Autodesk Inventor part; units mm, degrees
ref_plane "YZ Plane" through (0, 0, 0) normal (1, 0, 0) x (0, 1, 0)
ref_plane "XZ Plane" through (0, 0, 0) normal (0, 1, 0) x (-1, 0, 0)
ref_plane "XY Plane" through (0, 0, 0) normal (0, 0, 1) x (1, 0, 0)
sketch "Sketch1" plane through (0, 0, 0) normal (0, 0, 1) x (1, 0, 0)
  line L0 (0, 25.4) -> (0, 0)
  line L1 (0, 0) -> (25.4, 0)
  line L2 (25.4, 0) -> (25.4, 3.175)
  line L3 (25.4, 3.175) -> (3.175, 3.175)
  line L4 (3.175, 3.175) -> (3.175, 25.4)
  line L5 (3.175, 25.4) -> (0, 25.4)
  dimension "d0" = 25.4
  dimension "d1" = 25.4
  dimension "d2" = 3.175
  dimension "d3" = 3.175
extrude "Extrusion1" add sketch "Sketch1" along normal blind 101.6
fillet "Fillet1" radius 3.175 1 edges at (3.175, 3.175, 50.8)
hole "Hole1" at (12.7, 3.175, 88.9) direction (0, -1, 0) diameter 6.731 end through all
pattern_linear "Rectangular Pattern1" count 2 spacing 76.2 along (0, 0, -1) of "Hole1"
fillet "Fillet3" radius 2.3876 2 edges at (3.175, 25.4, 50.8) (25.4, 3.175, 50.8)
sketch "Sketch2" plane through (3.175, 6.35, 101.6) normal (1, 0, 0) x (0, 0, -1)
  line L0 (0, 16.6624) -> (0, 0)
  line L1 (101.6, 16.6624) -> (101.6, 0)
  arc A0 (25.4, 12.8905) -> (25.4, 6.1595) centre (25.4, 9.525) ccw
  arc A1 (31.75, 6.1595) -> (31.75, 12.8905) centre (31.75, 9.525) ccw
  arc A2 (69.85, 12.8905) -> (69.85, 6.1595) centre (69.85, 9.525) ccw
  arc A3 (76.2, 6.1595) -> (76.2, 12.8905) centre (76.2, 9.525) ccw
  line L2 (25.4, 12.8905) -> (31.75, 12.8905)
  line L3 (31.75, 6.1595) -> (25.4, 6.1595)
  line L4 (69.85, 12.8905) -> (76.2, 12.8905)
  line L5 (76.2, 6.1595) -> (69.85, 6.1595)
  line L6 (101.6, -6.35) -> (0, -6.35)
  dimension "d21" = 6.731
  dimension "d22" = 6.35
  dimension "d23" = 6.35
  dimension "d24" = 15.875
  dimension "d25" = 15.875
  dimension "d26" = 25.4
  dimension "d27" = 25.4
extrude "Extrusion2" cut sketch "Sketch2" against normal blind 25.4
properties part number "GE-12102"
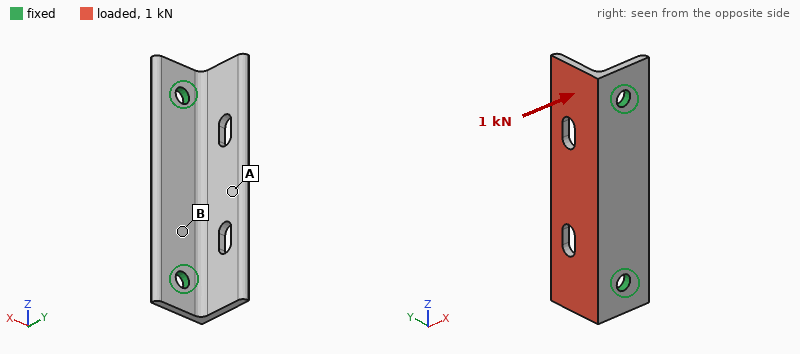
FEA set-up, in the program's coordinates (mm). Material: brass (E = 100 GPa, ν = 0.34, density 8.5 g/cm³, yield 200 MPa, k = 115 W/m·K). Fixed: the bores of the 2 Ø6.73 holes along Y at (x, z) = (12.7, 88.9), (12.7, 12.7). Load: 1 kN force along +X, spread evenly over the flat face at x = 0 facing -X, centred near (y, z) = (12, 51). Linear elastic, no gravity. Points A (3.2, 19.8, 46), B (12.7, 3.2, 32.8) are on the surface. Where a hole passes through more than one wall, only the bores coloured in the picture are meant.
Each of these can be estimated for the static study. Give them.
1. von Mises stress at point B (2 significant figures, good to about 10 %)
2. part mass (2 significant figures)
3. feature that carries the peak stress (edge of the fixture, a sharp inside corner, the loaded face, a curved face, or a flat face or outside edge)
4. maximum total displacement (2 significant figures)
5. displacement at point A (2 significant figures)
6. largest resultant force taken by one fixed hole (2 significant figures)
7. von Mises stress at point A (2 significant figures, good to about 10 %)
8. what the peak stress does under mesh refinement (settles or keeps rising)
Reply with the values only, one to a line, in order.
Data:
37 MPa
120 g
edge of the fixture
0.18 mm
0.13 mm
500 N
13 MPa
keeps rising
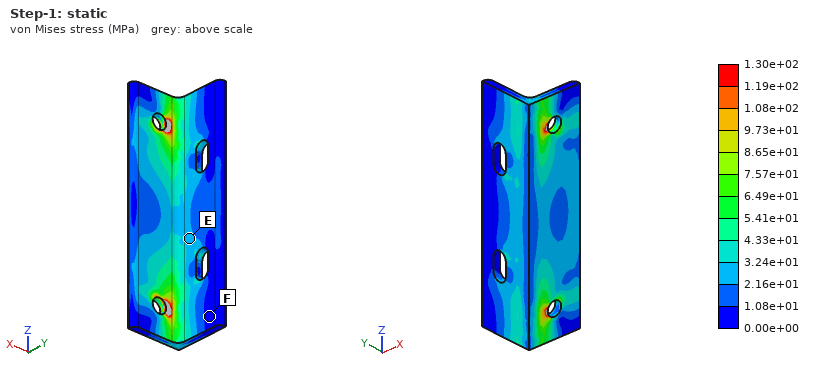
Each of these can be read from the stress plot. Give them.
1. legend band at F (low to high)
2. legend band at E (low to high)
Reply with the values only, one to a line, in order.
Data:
0.00e+00 to 1.08e+01 MPa
2.16e+01 to 3.24e+01 MPa
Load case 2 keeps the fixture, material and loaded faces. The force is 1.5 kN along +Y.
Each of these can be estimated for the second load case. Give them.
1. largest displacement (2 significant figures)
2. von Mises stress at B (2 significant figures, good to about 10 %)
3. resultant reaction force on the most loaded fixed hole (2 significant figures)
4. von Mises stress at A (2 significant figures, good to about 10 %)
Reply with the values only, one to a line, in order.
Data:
0.14 mm
26 MPa
790 N
14 MPa
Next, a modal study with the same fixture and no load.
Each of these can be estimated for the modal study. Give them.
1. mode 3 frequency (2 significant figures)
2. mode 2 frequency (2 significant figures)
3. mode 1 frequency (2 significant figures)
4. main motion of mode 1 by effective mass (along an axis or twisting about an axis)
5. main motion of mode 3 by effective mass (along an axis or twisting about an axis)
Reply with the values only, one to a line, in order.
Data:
3200 Hz
2600 Hz
1800 Hz
along X
along Y
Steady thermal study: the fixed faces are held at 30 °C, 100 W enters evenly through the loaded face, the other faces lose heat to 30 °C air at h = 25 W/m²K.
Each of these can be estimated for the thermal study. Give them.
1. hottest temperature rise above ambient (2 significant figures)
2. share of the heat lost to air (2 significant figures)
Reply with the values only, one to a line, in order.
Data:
88 K
8.7 %
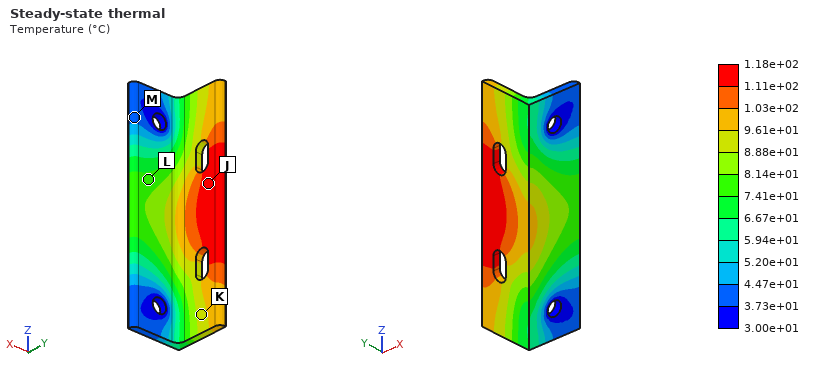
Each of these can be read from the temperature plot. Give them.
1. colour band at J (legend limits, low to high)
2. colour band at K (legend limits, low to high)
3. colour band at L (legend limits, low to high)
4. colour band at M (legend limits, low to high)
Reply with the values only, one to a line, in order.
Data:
1.11e+02 to 1.18e+02 °C
8.88e+01 to 9.61e+01 °C
7.41e+01 to 8.14e+01 °C
3.73e+01 to 4.47e+01 °C
